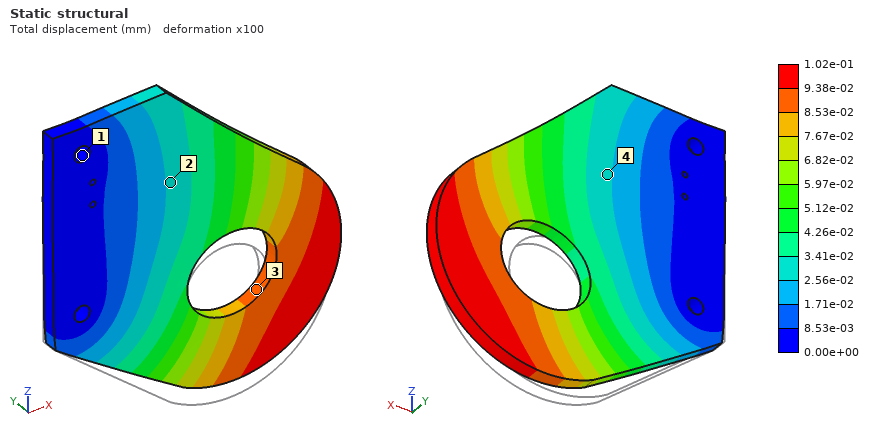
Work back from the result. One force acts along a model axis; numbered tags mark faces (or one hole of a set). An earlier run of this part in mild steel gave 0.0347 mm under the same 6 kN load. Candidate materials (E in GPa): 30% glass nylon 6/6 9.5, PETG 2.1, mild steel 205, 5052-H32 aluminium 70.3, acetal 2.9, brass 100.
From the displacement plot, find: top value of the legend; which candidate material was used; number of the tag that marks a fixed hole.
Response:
1.02e-01 mm
5052-H32 aluminium
1
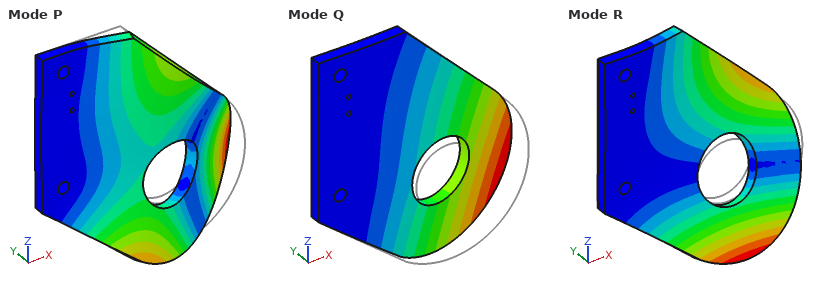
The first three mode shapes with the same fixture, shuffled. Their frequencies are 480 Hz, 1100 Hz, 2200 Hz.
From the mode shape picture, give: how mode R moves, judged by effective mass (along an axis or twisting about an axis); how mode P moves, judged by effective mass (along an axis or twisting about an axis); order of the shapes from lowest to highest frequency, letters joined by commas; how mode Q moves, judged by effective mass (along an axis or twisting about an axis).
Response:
twisting about X
along Y
Q, R, P
along Y
